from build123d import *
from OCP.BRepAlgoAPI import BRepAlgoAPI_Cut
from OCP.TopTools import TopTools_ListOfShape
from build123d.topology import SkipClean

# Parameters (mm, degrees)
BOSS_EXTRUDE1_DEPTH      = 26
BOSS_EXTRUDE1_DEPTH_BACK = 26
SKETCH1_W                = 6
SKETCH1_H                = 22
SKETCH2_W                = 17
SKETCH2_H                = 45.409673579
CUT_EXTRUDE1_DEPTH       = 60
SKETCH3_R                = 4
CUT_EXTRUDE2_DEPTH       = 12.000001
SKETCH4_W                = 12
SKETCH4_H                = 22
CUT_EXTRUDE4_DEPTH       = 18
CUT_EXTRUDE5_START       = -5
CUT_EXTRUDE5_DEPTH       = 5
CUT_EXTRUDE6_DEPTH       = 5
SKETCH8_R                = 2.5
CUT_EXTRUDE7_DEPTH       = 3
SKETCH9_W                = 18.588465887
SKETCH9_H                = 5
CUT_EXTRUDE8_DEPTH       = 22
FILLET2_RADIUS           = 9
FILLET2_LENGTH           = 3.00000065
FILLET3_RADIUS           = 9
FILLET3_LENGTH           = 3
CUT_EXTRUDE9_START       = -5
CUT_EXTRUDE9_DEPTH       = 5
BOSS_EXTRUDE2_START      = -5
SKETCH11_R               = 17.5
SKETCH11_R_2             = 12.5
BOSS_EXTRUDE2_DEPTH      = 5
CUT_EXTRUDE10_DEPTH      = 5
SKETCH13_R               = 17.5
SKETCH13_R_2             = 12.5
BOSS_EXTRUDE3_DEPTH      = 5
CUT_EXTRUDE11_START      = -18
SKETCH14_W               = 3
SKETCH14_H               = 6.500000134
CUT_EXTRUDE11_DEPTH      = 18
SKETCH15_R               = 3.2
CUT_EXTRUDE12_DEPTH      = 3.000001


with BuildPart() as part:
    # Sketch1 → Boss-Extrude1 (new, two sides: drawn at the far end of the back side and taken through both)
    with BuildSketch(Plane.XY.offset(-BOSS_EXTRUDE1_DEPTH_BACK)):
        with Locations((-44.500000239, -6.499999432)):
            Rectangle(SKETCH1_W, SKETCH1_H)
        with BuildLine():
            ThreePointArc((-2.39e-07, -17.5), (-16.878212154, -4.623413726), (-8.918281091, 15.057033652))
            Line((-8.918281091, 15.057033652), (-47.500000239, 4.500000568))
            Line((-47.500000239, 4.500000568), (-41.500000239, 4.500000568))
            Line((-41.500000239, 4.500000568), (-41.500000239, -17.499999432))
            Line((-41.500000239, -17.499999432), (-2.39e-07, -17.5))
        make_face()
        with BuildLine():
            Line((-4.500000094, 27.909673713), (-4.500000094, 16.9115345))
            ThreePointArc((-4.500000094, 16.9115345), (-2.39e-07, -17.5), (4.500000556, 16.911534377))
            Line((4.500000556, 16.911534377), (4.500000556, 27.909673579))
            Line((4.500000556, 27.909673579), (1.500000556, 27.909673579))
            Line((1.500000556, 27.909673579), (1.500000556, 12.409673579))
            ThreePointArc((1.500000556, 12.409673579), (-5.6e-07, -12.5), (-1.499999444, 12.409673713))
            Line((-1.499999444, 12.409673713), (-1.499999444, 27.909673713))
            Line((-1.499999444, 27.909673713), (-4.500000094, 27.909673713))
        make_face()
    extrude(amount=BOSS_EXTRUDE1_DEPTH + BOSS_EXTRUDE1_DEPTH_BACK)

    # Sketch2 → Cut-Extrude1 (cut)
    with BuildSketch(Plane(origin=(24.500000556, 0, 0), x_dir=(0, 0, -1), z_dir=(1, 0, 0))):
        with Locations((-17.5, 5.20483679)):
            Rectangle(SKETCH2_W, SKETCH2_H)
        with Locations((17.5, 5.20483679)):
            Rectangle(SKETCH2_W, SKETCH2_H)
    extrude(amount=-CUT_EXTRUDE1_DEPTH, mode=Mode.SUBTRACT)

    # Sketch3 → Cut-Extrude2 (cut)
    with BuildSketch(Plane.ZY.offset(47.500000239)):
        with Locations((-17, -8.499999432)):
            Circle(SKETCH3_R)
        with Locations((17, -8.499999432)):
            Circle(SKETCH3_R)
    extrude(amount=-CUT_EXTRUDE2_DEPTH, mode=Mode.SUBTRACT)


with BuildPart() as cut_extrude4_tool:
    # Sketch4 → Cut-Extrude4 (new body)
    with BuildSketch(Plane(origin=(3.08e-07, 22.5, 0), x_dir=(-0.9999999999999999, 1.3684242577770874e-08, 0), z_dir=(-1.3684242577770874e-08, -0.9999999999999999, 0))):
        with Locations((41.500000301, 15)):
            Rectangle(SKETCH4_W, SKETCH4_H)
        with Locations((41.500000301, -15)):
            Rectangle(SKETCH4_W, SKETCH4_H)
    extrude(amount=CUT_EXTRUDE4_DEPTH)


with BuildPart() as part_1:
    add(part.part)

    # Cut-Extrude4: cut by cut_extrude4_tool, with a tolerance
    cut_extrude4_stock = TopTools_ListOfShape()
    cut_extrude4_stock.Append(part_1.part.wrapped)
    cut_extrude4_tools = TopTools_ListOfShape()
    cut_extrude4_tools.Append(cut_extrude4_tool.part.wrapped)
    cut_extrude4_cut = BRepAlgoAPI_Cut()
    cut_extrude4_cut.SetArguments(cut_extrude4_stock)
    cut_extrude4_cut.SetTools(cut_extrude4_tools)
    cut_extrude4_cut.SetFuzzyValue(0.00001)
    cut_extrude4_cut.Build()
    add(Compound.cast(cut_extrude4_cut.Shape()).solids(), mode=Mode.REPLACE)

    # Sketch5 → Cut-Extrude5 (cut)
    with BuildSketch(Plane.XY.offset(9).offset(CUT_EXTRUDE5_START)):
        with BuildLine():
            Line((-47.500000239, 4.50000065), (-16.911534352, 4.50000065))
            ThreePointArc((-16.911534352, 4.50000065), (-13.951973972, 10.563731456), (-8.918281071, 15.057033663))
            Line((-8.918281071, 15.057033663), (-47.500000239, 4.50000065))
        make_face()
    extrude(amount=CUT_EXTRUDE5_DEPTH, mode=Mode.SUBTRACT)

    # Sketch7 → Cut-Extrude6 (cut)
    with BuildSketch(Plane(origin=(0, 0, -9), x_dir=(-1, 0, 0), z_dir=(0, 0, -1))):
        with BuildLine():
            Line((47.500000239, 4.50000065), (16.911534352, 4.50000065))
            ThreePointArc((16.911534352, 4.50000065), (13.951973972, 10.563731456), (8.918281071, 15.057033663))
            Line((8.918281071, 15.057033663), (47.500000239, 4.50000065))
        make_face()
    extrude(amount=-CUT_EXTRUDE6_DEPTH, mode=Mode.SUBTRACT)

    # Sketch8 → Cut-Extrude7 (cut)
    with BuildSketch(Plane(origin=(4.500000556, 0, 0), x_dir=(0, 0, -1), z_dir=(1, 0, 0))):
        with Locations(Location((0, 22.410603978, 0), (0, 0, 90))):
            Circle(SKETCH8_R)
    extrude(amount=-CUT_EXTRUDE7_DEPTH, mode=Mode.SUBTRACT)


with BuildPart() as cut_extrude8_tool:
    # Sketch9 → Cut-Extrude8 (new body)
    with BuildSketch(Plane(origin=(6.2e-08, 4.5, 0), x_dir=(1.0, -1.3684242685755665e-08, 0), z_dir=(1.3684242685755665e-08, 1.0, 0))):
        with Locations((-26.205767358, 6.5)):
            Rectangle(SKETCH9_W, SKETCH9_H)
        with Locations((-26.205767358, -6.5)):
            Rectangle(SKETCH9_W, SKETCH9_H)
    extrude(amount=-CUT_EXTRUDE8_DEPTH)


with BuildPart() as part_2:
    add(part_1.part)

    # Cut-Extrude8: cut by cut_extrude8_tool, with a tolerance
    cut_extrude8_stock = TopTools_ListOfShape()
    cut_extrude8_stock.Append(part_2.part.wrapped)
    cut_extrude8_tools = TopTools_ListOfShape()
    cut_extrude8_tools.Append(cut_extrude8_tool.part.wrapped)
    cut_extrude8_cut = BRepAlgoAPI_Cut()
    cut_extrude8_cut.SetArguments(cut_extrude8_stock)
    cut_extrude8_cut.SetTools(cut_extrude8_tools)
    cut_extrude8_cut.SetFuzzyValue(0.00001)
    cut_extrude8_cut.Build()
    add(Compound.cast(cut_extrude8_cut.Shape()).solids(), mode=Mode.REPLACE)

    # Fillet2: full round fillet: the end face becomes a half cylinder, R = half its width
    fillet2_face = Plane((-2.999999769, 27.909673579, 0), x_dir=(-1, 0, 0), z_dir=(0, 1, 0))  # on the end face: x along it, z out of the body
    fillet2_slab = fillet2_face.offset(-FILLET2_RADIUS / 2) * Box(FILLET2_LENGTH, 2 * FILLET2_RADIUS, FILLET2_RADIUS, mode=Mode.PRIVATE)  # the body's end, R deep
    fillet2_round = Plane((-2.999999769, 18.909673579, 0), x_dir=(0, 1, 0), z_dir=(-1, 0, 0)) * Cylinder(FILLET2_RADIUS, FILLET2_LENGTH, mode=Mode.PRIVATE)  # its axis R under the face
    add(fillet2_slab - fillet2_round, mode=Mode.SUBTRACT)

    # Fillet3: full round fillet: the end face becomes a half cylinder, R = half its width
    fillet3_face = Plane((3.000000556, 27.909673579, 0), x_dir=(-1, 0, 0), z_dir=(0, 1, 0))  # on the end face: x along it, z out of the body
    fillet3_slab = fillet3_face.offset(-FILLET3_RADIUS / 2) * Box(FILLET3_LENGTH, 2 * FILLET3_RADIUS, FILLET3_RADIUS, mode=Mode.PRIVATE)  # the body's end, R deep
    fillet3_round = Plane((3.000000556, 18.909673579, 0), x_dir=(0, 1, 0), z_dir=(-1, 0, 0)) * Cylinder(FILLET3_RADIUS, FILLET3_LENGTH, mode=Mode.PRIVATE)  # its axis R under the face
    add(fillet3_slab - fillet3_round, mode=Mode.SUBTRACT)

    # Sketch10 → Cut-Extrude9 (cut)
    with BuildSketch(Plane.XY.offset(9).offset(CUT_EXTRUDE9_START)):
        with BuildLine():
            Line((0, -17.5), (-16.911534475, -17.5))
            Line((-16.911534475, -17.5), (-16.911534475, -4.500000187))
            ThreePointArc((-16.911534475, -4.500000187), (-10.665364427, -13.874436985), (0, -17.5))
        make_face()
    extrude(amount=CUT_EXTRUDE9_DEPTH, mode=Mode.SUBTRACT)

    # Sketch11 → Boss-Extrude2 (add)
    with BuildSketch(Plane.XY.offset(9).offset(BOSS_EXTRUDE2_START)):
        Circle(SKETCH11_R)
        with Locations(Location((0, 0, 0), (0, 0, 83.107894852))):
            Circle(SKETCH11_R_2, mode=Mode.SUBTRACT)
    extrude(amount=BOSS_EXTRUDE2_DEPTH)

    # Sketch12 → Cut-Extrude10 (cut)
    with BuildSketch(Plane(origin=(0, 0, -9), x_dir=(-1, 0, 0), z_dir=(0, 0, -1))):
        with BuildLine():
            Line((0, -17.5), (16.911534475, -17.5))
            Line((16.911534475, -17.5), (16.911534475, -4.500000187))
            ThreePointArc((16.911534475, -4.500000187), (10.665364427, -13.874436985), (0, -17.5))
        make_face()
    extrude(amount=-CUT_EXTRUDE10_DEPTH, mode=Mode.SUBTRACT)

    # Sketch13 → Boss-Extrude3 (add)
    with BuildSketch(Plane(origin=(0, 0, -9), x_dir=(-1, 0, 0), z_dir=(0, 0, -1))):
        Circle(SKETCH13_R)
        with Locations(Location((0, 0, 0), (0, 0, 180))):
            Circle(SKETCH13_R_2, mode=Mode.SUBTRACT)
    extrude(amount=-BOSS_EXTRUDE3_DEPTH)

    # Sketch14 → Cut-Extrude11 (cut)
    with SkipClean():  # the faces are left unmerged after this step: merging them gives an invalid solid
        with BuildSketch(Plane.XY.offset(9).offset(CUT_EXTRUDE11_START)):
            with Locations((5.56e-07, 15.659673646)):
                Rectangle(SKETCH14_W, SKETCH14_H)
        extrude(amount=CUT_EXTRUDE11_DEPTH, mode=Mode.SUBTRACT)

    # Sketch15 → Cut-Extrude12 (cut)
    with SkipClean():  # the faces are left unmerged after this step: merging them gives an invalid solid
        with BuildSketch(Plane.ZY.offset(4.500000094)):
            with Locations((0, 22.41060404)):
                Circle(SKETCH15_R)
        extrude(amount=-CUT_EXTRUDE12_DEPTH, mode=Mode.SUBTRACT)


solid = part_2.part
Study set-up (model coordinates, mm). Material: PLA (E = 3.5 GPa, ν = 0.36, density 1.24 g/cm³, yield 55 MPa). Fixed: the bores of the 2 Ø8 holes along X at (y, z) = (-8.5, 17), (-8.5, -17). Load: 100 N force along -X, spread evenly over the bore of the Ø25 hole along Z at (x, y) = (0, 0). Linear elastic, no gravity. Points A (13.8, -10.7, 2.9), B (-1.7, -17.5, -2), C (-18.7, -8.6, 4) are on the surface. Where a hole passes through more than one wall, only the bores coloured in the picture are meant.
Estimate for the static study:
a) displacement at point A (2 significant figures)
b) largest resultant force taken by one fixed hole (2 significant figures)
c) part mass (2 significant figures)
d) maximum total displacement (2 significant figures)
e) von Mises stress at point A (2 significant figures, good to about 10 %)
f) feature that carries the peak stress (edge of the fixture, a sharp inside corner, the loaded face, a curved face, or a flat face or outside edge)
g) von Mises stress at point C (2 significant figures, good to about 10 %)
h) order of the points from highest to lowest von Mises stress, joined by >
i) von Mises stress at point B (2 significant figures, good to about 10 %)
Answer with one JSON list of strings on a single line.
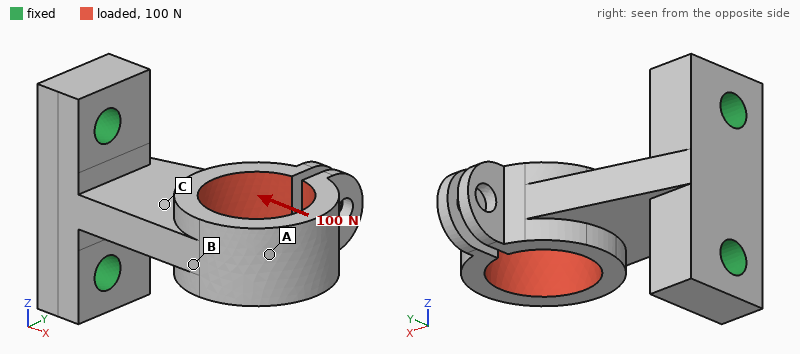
["0.32 mm", "51 N", "33 g", "1.1 mm", "4.8 MPa", "the loaded face", "1.3 MPa", "B > A > C", "8.3 MPa"]
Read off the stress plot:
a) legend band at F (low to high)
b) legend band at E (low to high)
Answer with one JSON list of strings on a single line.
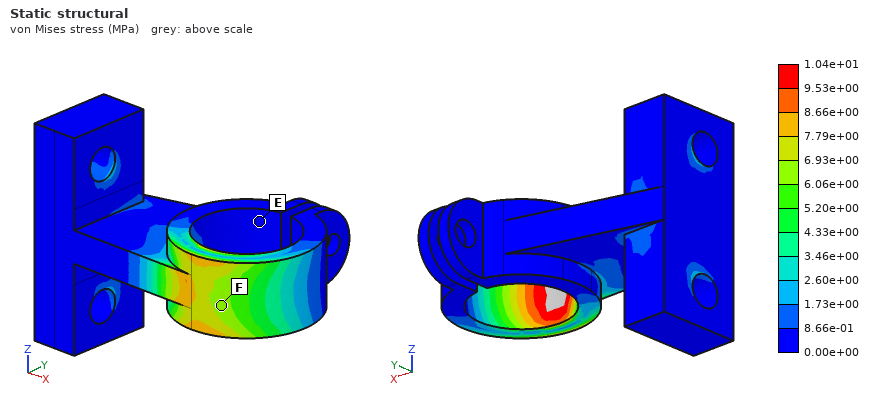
["6.06e+00 to 6.93e+00 MPa", "0.00e+00 to 8.66e-01 MPa"]
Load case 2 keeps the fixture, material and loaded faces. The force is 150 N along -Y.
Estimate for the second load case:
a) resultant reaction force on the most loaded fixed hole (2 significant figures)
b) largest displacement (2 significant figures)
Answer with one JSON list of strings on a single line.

["79 N", "0.94 mm"]
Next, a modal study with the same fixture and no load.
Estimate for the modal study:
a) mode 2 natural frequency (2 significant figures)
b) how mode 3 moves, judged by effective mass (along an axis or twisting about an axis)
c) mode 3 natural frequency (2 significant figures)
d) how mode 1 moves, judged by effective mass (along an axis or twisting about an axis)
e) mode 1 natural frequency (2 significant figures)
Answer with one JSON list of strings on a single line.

["490 Hz", "along Y", "960 Hz", "along Z", "470 Hz"]
